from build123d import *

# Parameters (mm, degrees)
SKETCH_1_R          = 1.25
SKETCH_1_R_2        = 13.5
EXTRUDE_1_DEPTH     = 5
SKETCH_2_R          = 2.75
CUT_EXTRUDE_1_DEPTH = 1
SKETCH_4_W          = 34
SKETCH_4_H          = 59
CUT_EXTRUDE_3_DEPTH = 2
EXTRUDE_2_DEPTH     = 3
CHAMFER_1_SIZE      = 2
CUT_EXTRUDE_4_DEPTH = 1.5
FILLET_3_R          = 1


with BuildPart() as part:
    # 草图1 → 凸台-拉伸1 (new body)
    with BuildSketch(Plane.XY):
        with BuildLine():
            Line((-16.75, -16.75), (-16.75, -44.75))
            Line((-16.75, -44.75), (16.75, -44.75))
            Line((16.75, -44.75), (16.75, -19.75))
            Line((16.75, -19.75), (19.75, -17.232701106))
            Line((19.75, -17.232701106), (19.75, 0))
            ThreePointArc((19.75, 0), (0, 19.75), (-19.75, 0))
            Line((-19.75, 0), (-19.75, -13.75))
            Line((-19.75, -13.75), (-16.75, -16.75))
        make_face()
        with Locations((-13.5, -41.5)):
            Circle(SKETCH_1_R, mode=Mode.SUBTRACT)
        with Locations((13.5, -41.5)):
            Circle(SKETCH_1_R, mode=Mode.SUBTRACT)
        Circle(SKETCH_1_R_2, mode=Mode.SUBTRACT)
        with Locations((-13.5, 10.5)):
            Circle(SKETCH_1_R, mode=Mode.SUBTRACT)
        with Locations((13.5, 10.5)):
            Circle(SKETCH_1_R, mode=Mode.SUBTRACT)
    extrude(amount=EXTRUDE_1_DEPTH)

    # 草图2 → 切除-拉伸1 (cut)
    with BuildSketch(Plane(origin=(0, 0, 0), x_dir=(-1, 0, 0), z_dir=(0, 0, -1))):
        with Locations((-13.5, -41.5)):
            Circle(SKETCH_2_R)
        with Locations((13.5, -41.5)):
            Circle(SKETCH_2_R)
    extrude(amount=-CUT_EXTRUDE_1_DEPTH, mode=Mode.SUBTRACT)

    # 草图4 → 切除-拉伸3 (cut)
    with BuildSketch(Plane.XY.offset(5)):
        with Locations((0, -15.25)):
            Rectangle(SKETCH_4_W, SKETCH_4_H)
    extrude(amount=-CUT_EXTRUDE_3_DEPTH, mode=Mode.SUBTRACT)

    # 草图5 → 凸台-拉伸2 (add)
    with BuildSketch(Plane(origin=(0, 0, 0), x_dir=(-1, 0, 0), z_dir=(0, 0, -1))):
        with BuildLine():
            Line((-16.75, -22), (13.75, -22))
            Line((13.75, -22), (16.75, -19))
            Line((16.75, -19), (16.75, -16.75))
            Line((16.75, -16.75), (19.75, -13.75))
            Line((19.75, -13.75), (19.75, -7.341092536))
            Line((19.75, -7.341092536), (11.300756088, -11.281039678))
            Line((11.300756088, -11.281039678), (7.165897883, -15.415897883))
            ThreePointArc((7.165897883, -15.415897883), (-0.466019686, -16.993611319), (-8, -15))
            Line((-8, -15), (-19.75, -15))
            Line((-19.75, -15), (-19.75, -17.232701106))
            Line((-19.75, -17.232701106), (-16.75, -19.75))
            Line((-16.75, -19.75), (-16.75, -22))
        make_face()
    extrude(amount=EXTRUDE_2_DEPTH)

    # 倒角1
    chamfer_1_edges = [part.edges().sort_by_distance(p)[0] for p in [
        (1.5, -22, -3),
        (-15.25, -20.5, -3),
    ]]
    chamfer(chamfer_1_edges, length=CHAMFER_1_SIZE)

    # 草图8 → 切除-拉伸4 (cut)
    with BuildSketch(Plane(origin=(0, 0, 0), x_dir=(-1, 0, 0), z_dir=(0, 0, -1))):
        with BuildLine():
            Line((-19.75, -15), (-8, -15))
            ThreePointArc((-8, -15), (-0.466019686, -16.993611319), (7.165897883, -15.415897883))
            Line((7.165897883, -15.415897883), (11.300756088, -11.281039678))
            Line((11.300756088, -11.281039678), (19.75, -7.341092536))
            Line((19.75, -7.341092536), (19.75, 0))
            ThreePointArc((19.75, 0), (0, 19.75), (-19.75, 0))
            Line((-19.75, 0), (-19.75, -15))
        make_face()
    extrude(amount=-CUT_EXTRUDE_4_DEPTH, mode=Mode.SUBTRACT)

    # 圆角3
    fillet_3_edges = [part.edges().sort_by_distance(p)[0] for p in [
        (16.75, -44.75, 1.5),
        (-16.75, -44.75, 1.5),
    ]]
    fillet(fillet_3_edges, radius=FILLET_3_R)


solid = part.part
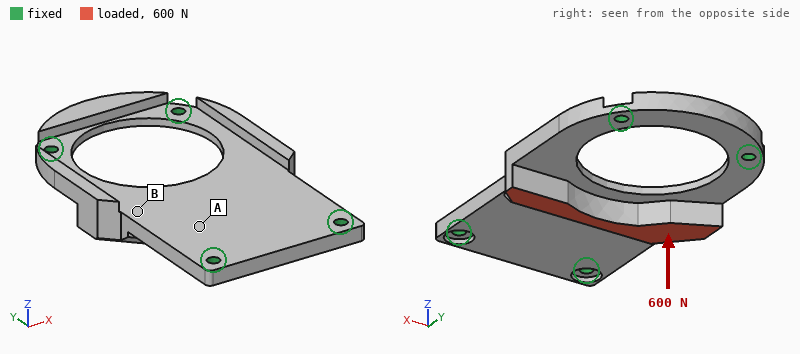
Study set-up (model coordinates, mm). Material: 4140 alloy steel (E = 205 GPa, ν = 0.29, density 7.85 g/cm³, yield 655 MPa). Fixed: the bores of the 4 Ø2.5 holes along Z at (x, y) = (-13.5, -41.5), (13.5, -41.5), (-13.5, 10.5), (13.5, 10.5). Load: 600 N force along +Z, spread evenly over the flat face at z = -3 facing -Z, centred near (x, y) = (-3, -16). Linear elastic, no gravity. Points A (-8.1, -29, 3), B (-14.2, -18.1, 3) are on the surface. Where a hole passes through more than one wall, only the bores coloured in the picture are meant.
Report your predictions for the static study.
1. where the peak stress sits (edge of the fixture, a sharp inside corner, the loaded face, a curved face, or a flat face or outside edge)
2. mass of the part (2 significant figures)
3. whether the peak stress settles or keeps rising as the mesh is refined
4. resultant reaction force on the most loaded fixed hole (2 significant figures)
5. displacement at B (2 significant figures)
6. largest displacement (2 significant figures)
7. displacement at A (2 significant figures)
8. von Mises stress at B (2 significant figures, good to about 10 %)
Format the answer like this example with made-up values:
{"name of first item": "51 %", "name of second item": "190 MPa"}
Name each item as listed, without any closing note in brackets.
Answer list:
{"where the peak stress sits": "edge of the fixture", "mass of the part": "41 g", "whether the peak stress settles or keeps rising as the mesh is refined": "keeps rising", "resultant reaction force on the most loaded fixed hole": "190 N", "displacement at B": "65 µm", "largest displacement": "80 µm", "displacement at A": "36 µm", "von Mises stress at B": "59 MPa"}
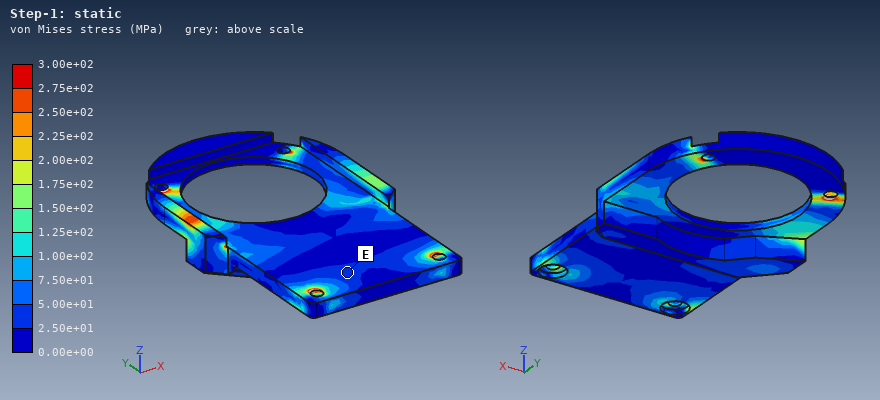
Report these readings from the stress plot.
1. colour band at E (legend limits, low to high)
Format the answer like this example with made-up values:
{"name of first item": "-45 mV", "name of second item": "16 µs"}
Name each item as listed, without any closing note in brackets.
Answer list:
{"colour band at E": "2.50e+01 to 5.00e+01 MPa"}
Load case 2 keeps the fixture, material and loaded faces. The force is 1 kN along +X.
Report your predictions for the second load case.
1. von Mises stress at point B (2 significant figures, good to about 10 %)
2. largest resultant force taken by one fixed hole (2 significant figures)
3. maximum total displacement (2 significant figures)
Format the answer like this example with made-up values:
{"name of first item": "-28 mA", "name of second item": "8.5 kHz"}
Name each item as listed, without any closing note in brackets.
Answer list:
{"von Mises stress at point B": "30 MPa", "largest resultant force taken by one fixed hole": "760 N", "maximum total displacement": "32 µm"}
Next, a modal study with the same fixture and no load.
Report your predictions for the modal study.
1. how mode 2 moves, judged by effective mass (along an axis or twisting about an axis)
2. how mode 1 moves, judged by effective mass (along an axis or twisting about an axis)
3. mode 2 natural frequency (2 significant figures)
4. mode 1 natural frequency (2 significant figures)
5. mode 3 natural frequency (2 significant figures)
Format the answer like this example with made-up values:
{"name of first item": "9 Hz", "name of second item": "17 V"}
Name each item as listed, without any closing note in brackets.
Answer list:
{"how mode 2 moves, judged by effective mass": "twisting about Y", "how mode 1 moves, judged by effective mass": "along Z", "mode 2 natural frequency": "4800 Hz", "mode 1 natural frequency": "3300 Hz", "mode 3 natural frequency": "7900 Hz"}
